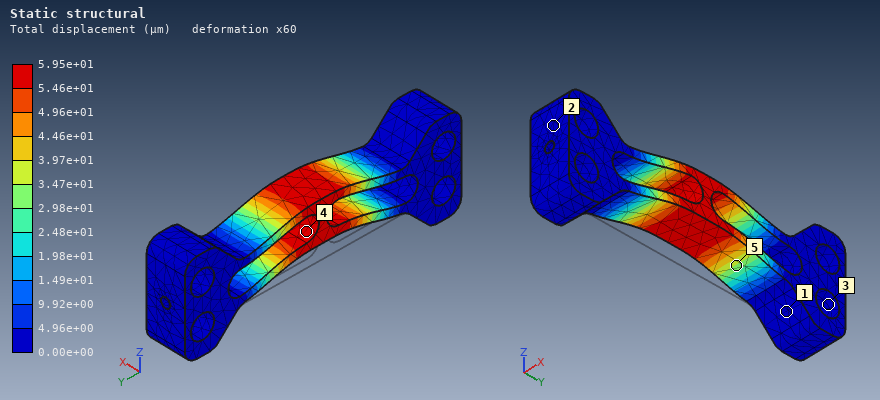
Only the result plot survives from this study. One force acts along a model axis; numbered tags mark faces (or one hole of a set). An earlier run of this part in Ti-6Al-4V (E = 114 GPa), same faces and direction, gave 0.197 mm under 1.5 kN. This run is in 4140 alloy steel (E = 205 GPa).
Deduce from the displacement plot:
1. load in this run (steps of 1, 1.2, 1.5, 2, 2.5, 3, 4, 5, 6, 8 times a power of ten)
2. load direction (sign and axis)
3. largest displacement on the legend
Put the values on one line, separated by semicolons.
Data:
800 N; +Z; 5.95e+01 µm
